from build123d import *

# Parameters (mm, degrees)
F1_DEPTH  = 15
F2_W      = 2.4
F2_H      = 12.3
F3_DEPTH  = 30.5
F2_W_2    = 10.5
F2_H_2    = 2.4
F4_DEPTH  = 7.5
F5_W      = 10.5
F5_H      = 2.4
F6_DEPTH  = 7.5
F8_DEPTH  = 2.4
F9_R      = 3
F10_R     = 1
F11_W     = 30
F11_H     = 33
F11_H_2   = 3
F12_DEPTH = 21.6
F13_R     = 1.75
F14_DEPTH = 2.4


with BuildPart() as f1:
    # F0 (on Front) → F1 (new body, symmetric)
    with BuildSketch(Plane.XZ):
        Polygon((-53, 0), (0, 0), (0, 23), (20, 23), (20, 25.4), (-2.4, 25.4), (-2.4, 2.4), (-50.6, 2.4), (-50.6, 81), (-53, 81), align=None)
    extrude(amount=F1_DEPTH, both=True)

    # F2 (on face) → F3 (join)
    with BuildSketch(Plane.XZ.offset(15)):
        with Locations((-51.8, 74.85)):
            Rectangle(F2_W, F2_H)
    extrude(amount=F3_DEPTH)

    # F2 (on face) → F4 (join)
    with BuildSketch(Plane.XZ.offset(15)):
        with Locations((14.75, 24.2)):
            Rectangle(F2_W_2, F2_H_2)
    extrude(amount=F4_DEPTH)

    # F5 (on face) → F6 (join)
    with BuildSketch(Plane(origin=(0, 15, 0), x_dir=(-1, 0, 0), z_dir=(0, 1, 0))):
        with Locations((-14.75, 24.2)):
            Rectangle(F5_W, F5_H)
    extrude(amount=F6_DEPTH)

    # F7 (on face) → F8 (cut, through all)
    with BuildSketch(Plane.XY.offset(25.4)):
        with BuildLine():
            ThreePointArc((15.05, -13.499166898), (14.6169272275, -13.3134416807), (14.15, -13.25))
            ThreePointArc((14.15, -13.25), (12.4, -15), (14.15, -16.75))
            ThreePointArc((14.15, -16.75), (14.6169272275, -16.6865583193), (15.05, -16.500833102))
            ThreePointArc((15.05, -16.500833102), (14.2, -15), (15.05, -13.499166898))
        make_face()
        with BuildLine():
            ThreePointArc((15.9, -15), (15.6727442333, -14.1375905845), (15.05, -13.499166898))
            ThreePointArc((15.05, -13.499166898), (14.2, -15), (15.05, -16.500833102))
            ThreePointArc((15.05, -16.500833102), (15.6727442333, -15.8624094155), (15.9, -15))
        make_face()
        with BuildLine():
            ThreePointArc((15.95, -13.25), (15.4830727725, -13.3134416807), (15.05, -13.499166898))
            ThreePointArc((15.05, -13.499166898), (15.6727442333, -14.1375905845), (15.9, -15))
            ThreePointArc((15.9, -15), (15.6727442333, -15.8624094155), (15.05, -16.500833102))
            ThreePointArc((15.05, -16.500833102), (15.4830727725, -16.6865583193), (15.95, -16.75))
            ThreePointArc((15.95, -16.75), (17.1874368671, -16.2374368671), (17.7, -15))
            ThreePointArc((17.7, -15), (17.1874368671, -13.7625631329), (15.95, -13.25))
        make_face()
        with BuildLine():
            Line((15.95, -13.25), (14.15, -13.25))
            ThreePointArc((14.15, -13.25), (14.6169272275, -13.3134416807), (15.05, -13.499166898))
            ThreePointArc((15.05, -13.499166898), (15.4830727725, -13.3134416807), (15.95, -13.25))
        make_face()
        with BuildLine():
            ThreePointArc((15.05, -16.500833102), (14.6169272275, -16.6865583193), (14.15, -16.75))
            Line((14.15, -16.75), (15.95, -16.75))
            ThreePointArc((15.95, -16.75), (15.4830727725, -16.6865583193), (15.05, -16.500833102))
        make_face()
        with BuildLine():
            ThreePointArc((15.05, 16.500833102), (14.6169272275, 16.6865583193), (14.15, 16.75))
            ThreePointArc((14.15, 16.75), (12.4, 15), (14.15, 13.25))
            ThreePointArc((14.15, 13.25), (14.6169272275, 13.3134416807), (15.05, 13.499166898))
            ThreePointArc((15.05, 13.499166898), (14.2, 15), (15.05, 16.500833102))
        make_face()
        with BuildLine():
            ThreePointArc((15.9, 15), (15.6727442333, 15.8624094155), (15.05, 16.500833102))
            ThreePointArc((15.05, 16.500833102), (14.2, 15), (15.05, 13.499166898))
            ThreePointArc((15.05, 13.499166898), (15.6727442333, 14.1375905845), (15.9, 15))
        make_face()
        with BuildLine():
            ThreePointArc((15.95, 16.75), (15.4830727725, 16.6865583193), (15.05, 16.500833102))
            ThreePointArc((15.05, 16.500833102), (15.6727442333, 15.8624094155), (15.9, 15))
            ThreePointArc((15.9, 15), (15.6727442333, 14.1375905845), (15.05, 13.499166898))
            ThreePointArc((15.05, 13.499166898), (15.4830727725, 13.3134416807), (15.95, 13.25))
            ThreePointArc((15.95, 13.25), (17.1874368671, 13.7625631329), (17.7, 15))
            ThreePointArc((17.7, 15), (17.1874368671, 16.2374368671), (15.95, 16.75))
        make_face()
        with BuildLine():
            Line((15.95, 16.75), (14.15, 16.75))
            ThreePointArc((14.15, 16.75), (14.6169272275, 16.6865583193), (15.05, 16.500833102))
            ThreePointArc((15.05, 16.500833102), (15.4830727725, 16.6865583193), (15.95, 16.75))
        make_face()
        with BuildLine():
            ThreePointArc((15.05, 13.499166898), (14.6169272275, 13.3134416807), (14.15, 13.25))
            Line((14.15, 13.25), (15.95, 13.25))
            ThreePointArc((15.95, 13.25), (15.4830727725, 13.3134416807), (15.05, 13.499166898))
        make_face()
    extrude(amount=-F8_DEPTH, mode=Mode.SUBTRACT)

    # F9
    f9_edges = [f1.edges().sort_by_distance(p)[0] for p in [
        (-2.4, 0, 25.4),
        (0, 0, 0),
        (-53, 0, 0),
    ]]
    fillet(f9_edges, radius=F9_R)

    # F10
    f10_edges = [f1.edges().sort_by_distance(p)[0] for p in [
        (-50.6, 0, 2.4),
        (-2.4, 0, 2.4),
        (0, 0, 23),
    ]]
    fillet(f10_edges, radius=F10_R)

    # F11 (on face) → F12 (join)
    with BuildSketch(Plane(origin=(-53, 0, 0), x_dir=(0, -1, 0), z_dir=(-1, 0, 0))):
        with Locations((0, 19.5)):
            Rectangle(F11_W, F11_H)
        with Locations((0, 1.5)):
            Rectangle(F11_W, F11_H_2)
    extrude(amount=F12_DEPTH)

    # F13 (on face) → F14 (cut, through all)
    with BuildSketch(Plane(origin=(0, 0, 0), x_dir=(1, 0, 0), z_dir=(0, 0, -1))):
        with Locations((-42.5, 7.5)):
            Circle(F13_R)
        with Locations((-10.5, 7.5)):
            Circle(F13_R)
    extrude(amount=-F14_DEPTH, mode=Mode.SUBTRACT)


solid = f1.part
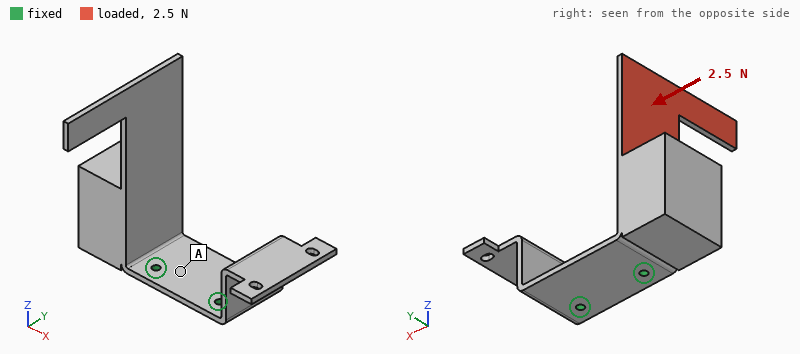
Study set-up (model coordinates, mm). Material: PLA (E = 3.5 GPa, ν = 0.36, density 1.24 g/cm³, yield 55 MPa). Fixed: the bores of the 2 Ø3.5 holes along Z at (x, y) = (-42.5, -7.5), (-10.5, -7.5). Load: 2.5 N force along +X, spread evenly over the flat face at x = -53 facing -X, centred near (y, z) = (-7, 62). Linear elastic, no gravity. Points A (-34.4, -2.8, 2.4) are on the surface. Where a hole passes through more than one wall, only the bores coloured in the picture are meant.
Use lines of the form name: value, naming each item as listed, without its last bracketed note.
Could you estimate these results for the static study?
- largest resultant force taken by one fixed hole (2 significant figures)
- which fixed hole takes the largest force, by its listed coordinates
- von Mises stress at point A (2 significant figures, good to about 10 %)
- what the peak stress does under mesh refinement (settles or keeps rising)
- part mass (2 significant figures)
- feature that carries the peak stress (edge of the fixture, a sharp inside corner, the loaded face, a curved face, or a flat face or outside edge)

largest resultant force taken by one fixed hole: 2.7 N
which fixed hole takes the largest force, by its listed coordinates: (-42.5, -7.5)
von Mises stress at point A: 0.63 MPa
what the peak stress does under mesh refinement: keeps rising
part mass: 46 g
feature that carries the peak stress: edge of the fixture
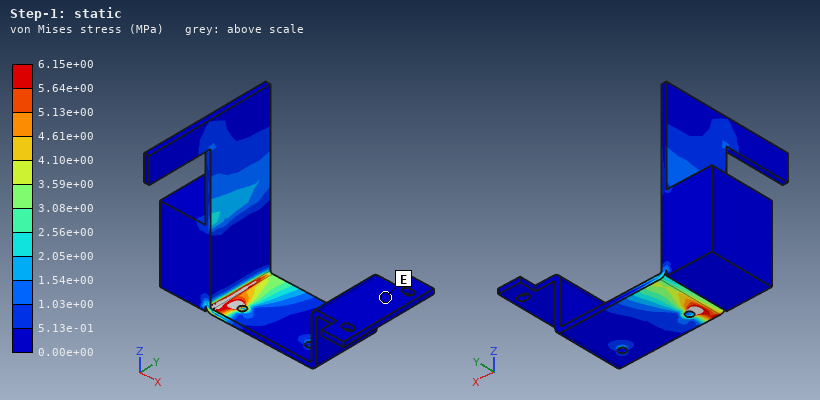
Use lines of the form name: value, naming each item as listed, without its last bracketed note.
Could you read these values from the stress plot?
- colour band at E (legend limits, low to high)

colour band at E: 0.00e+00 to 5.13e-01 MPa
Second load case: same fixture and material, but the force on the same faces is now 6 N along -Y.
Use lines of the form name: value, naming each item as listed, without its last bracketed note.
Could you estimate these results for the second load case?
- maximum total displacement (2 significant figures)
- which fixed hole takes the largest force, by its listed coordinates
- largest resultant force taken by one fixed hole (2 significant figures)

maximum total displacement: 1.5 mm
which fixed hole takes the largest force, by its listed coordinates: (-42.5, -7.5)
largest resultant force taken by one fixed hole: 7.3 N
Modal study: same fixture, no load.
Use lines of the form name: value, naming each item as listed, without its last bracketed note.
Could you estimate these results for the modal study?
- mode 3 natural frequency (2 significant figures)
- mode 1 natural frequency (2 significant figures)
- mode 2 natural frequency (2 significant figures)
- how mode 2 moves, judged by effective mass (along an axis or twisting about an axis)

mode 3 natural frequency: 260 Hz
mode 1 natural frequency: 76 Hz
mode 2 natural frequency: 130 Hz
how mode 2 moves, judged by effective mass: along Y
